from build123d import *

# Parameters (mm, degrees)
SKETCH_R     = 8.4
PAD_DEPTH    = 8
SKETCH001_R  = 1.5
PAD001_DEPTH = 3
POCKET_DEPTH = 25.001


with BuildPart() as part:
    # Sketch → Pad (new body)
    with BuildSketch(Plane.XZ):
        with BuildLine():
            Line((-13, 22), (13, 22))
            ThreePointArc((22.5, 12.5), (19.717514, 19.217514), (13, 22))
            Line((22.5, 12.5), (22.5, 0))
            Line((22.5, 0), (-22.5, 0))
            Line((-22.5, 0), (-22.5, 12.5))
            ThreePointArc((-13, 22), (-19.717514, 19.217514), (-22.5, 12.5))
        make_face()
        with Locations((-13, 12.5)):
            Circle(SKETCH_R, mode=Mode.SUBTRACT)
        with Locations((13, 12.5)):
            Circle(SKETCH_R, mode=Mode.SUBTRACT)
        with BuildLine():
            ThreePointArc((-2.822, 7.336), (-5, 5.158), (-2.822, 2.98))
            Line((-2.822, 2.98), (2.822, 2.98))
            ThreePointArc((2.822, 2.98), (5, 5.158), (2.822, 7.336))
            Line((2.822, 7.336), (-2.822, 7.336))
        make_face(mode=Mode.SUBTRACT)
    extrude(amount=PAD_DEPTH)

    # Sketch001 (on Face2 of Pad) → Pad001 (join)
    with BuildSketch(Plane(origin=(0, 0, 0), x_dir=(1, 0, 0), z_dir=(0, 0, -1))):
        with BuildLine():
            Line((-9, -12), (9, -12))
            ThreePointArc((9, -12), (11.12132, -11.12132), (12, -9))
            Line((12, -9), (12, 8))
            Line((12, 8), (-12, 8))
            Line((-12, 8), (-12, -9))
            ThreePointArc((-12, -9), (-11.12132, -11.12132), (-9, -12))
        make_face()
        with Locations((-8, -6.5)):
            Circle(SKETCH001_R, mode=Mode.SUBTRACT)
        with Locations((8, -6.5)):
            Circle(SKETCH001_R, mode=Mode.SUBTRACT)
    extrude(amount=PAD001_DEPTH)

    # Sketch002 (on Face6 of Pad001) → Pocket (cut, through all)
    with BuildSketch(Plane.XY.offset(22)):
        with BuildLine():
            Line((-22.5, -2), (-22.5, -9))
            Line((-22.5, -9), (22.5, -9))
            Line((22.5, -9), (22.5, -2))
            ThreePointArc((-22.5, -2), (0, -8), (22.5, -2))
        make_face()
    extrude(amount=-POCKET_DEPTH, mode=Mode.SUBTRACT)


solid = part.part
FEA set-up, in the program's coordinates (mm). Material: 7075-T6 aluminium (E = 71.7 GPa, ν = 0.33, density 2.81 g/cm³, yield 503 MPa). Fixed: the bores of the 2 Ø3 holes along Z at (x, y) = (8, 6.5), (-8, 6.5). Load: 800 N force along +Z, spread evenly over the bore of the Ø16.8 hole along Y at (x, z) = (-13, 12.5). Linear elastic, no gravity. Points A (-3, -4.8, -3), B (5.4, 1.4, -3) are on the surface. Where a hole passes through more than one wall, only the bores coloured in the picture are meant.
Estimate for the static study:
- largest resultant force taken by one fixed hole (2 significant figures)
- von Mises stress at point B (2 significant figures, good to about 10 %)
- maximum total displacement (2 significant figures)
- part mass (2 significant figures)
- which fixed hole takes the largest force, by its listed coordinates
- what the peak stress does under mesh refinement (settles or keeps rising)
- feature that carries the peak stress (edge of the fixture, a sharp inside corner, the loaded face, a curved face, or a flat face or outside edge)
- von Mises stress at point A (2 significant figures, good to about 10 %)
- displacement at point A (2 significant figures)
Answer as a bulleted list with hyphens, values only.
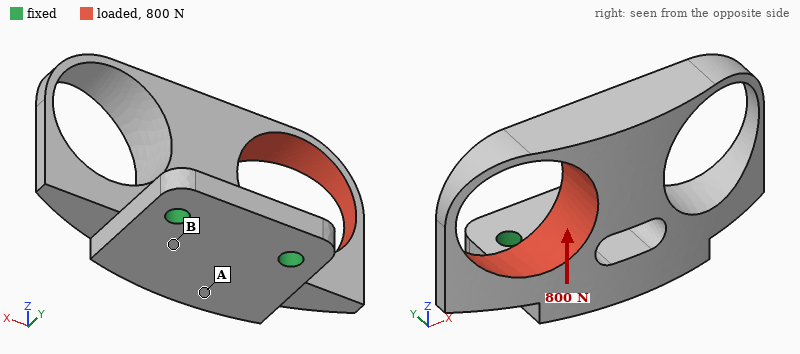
- 900 N
- 97 MPa
- 0.29 mm
- 12 g
- (-8, 6.5)
- keeps rising
- edge of the fixture
- 37 MPa
- 0.082 mm
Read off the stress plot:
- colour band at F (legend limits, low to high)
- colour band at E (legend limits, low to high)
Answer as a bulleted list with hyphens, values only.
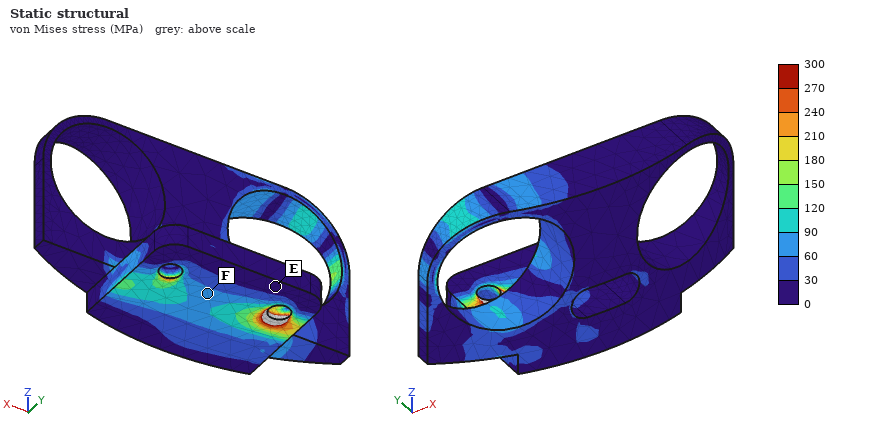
- 60 to 90 MPa
- 0 to 30 MPa
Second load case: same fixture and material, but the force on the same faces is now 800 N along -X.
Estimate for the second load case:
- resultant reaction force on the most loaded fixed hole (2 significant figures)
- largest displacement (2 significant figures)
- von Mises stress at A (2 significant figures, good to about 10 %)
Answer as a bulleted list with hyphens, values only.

- 860 N
- 0.14 mm
- 34 MPa
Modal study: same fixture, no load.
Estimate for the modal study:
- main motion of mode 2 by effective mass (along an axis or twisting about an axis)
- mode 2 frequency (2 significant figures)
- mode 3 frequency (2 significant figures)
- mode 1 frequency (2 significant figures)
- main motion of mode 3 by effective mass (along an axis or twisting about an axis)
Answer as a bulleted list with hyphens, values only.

- along X
- 5600 Hz
- 10000 Hz
- 2400 Hz
- along Z
